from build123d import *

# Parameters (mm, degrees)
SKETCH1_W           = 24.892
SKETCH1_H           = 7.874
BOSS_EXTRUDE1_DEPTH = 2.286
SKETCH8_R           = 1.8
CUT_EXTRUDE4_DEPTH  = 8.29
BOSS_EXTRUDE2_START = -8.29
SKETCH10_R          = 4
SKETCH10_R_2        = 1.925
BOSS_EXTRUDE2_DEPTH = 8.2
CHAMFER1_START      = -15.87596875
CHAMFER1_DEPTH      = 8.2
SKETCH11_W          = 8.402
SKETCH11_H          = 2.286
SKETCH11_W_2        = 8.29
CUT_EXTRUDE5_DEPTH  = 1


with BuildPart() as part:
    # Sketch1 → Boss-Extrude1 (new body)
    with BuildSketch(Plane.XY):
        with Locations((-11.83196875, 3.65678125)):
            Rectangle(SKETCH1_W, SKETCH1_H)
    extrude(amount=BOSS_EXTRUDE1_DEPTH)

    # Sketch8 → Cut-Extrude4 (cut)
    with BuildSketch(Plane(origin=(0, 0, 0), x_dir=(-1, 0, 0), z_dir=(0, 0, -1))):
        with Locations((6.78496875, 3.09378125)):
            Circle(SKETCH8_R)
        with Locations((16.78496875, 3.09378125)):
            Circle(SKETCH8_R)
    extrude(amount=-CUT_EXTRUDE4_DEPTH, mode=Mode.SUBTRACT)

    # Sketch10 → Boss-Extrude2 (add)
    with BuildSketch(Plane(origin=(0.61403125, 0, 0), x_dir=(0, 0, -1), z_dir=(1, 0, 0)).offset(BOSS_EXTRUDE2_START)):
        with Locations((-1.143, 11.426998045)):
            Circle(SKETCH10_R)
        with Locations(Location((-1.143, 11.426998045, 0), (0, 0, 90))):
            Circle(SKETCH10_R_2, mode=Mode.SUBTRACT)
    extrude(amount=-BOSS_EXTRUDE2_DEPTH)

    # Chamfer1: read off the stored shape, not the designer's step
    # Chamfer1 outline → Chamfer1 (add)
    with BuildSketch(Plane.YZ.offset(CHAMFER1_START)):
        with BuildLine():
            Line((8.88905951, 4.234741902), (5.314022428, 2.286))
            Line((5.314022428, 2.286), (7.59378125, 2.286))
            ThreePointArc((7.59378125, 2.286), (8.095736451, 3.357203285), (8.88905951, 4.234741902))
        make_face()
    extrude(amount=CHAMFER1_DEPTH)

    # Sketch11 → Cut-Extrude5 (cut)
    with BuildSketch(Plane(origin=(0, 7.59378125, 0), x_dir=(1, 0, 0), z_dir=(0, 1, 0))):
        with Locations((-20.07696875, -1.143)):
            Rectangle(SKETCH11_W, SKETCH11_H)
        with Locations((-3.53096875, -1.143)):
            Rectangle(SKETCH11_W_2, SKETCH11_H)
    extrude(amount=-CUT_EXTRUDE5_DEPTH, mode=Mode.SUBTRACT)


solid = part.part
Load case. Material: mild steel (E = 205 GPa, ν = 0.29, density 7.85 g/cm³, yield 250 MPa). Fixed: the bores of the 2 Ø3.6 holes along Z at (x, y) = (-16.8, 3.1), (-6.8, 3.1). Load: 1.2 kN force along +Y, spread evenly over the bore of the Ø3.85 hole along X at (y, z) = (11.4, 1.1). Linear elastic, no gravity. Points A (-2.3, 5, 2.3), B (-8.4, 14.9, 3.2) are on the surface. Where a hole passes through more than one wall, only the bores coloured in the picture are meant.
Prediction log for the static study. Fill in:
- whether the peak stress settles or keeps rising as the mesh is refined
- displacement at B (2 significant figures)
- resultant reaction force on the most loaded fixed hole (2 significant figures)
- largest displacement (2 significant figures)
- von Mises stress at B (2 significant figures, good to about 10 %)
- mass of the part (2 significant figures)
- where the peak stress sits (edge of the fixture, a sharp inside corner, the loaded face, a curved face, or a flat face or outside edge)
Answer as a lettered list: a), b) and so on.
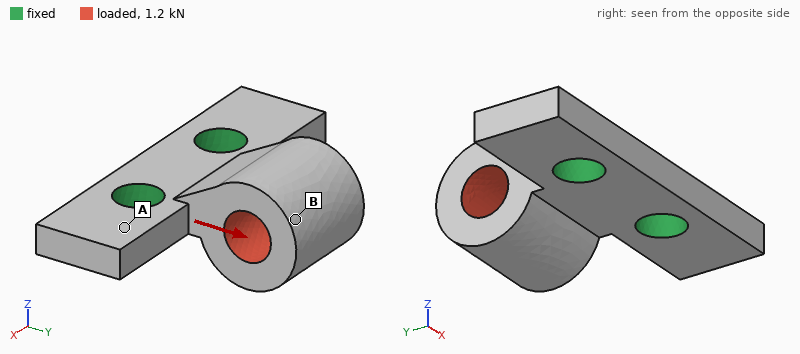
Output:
a) keeps rising
b) 3.8 µm
c) 640 N
d) 4.8 µm
e) 21 MPa
f) 5.4 g
g) a sharp inside corner
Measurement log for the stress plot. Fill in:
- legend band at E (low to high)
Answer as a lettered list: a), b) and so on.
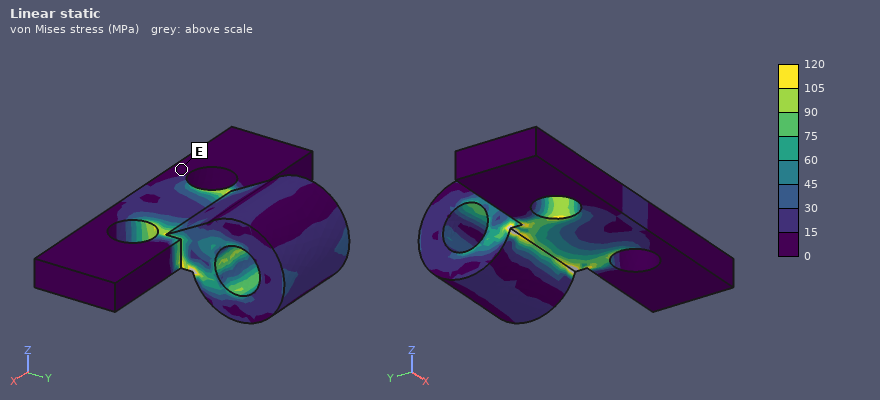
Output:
a) 0 to 15 MPa
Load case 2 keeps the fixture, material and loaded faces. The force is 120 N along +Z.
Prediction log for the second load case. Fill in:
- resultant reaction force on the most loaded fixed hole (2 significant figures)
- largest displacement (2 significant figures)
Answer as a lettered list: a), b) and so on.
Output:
a) 60 N
b) 12 µm
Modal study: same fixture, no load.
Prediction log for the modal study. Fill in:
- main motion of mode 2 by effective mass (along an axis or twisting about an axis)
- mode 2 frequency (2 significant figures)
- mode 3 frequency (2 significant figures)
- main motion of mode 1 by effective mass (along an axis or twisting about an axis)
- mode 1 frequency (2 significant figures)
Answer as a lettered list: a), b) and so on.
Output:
a) along X
b) 34 kHz
c) 45 kHz
d) along Z
e) 11 kHz
